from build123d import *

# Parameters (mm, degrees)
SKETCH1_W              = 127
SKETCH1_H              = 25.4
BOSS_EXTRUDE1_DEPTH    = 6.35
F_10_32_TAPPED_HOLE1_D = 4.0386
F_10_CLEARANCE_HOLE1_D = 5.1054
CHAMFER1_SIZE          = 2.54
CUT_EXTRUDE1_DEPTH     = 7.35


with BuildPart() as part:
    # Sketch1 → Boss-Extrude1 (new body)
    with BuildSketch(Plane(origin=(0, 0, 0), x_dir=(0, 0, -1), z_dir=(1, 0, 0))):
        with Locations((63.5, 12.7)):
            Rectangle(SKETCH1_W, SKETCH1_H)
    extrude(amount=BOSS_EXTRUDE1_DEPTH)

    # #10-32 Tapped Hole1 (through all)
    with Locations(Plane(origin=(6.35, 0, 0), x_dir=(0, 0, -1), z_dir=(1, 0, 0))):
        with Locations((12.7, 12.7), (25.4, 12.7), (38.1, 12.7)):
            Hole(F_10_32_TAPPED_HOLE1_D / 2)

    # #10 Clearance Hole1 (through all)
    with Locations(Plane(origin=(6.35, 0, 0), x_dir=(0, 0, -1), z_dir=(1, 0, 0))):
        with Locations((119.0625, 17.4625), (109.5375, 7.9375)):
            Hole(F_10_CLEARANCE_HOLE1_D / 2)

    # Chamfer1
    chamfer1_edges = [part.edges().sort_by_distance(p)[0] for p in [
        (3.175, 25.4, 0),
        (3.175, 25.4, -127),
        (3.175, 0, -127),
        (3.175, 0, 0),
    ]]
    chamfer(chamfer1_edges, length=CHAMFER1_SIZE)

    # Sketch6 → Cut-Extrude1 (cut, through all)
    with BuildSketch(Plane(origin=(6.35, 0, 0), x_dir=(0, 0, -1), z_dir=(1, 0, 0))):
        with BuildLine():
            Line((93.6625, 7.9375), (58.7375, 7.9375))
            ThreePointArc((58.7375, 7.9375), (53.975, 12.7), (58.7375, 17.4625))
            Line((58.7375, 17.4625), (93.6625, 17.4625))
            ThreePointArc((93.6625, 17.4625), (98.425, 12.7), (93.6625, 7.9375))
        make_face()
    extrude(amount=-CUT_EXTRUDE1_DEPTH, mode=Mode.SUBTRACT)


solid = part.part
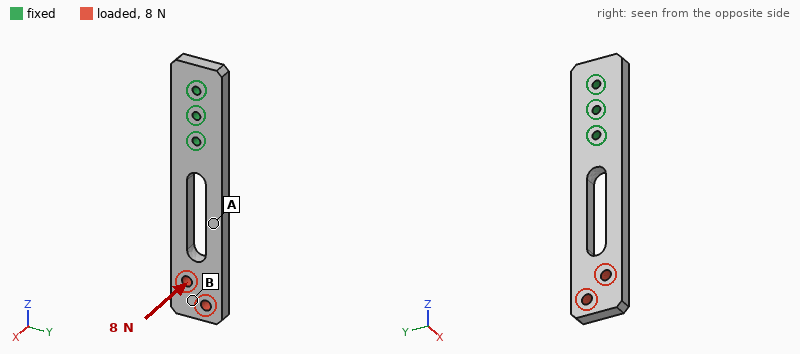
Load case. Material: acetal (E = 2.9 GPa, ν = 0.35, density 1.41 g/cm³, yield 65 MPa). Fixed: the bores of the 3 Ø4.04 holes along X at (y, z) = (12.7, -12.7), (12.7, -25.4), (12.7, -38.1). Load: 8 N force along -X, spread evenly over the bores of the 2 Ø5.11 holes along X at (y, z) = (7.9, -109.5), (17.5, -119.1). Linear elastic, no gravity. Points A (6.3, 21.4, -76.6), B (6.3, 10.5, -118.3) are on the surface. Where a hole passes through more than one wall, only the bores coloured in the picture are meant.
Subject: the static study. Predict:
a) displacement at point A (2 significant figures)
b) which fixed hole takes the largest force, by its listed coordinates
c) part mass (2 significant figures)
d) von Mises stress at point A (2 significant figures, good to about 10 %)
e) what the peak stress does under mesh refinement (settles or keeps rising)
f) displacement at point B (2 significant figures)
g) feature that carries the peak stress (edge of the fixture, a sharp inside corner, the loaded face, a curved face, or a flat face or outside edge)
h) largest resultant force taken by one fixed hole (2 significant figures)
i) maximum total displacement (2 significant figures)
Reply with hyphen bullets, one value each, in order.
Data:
- 0.30 mm
- (12.7, -38.1)
- 24 g
- 2.8 MPa
- keeps rising
- 1.1 mm
- edge of the fixture
- 27 N
- 1.3 mm
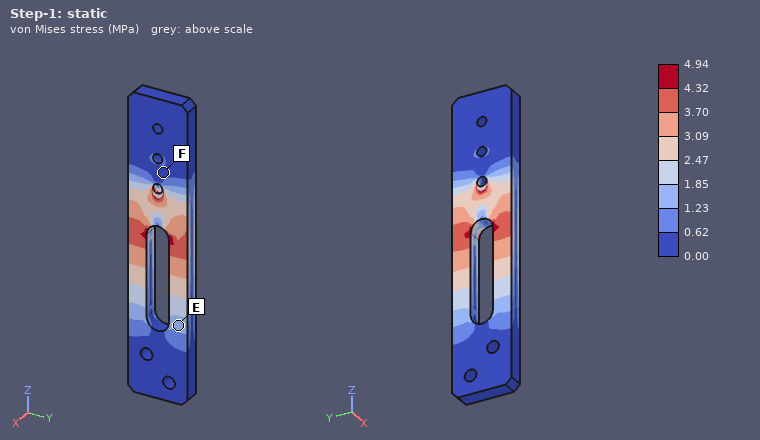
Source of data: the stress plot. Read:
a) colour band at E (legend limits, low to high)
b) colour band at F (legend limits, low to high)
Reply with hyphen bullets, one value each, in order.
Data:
- 1.23 to 1.85 MPa
- 0.00 to 0.62 MPa
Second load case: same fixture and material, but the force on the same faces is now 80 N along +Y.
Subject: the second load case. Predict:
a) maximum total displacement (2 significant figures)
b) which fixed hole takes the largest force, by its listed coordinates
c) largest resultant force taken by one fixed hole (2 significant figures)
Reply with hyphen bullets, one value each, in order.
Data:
- 1.4 mm
- (12.7, -38.1)
- 330 N
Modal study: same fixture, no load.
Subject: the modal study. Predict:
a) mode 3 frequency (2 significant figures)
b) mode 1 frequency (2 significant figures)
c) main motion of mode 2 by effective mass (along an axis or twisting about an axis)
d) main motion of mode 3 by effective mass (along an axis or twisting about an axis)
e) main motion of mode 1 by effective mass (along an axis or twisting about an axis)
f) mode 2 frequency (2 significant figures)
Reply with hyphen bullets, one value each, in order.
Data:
- 850 Hz
- 170 Hz
- along Y
- twisting about Z
- along X
- 470 Hz
